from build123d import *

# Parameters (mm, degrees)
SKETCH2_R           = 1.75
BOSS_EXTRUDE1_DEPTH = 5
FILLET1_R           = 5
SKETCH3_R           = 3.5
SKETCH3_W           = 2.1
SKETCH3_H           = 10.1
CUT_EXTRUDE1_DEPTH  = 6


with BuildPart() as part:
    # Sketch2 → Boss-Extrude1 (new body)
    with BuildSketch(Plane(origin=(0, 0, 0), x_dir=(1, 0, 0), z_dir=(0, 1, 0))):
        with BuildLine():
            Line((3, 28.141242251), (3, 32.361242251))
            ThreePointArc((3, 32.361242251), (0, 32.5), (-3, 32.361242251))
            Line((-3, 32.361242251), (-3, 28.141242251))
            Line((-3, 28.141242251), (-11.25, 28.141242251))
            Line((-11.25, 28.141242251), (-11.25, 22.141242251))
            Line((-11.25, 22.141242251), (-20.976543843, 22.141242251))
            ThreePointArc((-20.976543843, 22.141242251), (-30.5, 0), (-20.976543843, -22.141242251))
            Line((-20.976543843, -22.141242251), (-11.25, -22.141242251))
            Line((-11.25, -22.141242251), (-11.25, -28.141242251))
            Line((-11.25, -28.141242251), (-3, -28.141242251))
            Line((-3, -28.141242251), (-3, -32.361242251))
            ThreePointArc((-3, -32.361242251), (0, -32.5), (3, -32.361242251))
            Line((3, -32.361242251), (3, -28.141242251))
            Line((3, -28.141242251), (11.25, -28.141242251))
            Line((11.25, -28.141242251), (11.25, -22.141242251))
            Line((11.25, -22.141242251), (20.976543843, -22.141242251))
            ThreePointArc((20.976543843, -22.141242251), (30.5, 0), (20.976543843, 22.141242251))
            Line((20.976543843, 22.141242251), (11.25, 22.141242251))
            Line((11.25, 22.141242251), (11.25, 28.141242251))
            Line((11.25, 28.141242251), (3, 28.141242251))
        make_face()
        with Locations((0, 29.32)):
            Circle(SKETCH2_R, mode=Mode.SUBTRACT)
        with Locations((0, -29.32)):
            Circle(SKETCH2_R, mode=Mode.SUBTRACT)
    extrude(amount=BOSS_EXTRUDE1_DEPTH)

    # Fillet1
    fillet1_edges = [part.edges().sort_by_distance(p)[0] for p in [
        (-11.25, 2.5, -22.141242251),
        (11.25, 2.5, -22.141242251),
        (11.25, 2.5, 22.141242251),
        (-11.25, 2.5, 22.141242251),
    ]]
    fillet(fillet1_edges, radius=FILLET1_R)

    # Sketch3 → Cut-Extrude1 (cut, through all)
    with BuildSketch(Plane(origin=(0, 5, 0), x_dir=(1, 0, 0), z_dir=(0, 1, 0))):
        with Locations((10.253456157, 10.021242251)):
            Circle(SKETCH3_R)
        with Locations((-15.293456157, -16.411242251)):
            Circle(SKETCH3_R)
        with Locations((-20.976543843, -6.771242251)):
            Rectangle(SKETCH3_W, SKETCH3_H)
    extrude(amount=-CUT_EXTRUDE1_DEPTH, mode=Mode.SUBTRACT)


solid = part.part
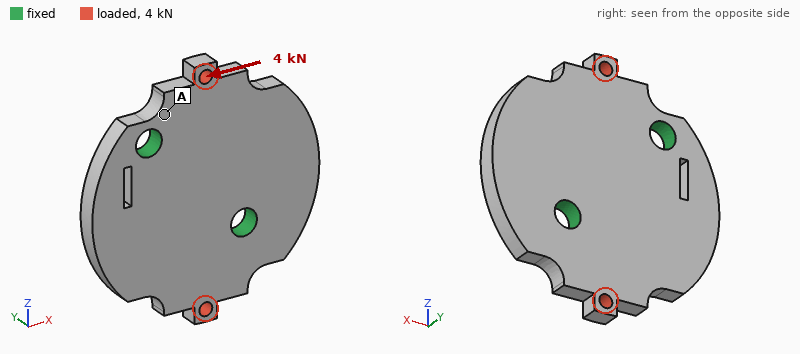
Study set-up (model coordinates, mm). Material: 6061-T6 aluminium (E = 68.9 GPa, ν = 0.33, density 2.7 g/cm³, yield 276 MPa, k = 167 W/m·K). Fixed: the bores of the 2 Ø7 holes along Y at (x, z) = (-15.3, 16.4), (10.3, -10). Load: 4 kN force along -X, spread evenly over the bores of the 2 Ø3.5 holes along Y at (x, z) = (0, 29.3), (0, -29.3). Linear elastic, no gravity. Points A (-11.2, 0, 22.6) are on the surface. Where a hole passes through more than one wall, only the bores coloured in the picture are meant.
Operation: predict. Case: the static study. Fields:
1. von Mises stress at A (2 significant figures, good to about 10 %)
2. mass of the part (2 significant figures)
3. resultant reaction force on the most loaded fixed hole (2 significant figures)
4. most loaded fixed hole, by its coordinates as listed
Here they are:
40 MPa
36 g
2.3 kN
(10.3, -10)
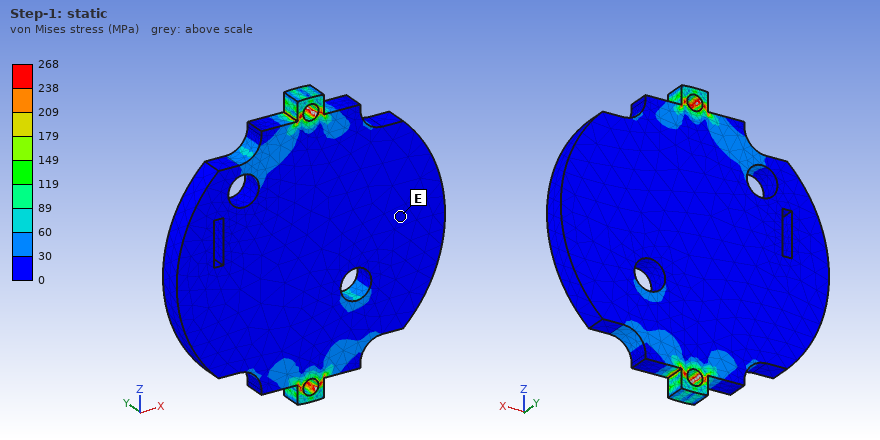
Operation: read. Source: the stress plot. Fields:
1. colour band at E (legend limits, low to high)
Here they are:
0 to 30 MPa
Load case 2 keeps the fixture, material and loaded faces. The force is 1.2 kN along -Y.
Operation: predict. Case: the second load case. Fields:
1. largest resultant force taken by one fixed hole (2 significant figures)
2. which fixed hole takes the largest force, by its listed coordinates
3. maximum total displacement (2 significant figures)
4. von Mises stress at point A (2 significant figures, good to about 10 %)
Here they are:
660 N
(10.3, -10)
0.12 mm
90 MPa
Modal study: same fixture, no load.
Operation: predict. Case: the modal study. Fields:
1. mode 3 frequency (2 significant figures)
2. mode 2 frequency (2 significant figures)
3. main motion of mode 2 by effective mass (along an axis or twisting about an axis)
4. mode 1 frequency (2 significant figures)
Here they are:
11 kHz
6300 Hz
along Y
5300 Hz
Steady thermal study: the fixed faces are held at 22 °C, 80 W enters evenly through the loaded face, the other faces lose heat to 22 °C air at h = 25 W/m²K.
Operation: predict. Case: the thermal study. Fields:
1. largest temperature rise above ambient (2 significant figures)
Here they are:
80 K
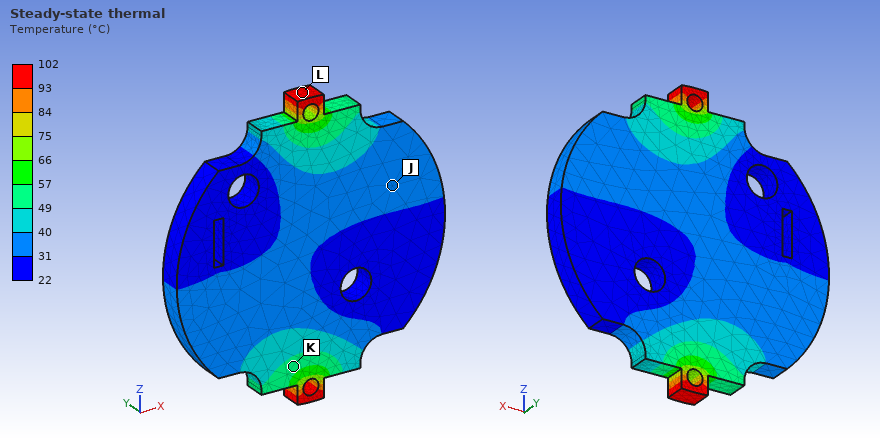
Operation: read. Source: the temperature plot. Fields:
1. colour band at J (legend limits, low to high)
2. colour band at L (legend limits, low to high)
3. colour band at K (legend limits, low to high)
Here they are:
31 to 40 °C
93 to 102 °C
49 to 57 °C
